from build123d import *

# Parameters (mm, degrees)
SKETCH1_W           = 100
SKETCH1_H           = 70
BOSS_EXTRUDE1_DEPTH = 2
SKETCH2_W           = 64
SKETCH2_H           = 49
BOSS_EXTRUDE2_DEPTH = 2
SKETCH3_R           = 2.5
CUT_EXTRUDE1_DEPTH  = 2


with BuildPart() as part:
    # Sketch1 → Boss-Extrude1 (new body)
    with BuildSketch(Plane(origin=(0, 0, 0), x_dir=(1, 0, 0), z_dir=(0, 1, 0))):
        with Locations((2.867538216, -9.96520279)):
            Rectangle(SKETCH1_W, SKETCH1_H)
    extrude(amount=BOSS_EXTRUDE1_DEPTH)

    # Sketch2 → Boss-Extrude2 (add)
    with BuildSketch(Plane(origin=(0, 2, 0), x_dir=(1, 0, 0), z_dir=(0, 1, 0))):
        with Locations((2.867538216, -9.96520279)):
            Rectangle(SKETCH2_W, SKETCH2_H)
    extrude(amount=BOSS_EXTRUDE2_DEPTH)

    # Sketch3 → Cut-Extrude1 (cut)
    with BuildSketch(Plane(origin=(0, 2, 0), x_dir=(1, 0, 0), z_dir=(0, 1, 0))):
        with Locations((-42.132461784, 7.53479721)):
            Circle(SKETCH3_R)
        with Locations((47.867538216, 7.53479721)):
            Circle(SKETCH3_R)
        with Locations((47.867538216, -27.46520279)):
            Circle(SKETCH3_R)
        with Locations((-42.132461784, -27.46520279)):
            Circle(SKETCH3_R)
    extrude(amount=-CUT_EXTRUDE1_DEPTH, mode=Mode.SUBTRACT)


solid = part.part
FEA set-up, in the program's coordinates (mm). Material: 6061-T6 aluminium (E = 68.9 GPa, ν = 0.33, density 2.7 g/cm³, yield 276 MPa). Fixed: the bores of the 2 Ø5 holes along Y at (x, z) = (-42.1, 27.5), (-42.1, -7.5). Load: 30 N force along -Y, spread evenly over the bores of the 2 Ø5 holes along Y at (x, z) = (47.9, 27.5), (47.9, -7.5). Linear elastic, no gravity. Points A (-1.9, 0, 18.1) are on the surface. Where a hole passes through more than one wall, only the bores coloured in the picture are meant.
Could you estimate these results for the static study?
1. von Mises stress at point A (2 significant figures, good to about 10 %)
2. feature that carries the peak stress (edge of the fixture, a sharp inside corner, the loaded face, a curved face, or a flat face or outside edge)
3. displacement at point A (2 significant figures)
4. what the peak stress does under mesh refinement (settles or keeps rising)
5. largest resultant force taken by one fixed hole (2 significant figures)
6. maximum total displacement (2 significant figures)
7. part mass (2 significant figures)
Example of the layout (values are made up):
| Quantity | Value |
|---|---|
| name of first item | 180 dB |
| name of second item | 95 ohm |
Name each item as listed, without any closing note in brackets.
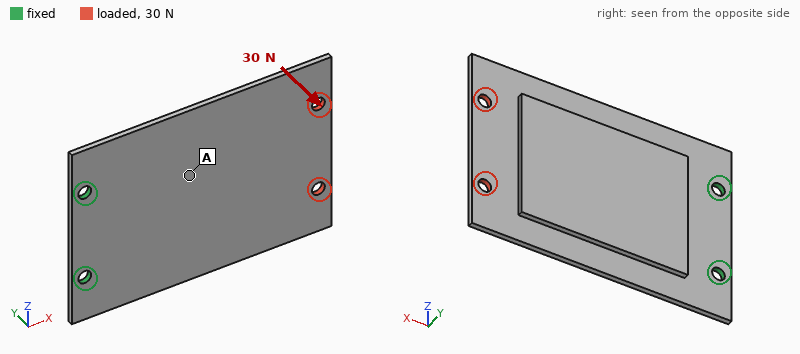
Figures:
| Quantity | Value |
|---|---|
| von Mises stress at point A | 10 MPa |
| feature that carries the peak stress | edge of the fixture |
| displacement at point A | 0.42 mm |
| what the peak stress does under mesh refinement | keeps rising |
| largest resultant force taken by one fixed hole | 31 N |
| maximum total displacement | 1.2 mm |
| part mass | 54 g |
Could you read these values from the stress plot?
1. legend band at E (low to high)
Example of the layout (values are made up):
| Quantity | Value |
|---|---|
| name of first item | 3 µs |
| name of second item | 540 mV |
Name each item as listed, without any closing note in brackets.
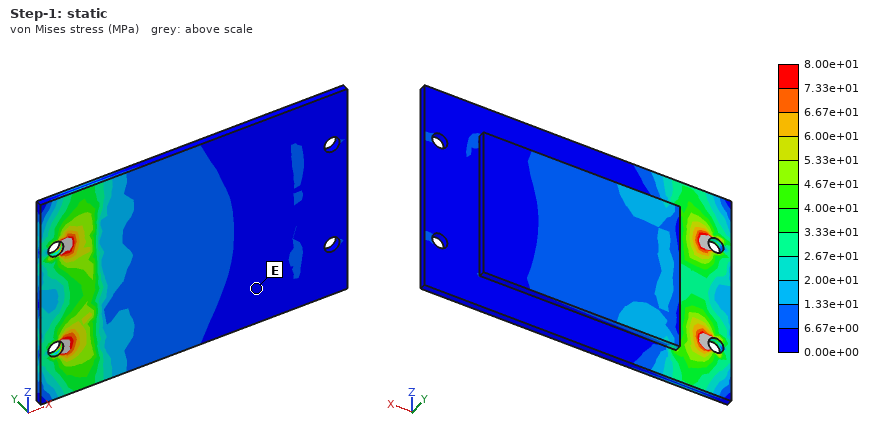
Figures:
| Quantity | Value |
|---|---|
| legend band at E | 0.00e+00 to 6.67e+00 MPa |
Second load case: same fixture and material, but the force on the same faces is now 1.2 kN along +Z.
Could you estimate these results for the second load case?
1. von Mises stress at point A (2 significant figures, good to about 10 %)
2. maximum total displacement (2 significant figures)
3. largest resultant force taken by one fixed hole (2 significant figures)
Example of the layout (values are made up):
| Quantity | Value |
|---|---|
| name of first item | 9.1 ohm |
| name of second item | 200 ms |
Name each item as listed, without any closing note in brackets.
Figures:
| Quantity | Value |
|---|---|
| von Mises stress at point A | 26 MPa |
| maximum total displacement | 0.30 mm |
| largest resultant force taken by one fixed hole | 2.9 kN |
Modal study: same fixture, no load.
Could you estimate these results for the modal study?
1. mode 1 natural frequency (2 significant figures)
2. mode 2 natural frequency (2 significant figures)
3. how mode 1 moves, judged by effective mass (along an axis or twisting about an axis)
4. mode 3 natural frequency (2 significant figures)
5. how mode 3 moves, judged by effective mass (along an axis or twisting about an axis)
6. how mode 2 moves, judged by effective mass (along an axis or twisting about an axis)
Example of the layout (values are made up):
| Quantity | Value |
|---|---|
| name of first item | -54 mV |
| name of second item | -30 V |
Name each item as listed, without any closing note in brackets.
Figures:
| Quantity | Value |
|---|---|
| mode 1 natural frequency | 210 Hz |
| mode 2 natural frequency | 970 Hz |
| how mode 1 moves, judged by effective mass | along Y |
| mode 3 natural frequency | 1900 Hz |
| how mode 3 moves, judged by effective mass | along Y |
| how mode 2 moves, judged by effective mass | twisting about X |
